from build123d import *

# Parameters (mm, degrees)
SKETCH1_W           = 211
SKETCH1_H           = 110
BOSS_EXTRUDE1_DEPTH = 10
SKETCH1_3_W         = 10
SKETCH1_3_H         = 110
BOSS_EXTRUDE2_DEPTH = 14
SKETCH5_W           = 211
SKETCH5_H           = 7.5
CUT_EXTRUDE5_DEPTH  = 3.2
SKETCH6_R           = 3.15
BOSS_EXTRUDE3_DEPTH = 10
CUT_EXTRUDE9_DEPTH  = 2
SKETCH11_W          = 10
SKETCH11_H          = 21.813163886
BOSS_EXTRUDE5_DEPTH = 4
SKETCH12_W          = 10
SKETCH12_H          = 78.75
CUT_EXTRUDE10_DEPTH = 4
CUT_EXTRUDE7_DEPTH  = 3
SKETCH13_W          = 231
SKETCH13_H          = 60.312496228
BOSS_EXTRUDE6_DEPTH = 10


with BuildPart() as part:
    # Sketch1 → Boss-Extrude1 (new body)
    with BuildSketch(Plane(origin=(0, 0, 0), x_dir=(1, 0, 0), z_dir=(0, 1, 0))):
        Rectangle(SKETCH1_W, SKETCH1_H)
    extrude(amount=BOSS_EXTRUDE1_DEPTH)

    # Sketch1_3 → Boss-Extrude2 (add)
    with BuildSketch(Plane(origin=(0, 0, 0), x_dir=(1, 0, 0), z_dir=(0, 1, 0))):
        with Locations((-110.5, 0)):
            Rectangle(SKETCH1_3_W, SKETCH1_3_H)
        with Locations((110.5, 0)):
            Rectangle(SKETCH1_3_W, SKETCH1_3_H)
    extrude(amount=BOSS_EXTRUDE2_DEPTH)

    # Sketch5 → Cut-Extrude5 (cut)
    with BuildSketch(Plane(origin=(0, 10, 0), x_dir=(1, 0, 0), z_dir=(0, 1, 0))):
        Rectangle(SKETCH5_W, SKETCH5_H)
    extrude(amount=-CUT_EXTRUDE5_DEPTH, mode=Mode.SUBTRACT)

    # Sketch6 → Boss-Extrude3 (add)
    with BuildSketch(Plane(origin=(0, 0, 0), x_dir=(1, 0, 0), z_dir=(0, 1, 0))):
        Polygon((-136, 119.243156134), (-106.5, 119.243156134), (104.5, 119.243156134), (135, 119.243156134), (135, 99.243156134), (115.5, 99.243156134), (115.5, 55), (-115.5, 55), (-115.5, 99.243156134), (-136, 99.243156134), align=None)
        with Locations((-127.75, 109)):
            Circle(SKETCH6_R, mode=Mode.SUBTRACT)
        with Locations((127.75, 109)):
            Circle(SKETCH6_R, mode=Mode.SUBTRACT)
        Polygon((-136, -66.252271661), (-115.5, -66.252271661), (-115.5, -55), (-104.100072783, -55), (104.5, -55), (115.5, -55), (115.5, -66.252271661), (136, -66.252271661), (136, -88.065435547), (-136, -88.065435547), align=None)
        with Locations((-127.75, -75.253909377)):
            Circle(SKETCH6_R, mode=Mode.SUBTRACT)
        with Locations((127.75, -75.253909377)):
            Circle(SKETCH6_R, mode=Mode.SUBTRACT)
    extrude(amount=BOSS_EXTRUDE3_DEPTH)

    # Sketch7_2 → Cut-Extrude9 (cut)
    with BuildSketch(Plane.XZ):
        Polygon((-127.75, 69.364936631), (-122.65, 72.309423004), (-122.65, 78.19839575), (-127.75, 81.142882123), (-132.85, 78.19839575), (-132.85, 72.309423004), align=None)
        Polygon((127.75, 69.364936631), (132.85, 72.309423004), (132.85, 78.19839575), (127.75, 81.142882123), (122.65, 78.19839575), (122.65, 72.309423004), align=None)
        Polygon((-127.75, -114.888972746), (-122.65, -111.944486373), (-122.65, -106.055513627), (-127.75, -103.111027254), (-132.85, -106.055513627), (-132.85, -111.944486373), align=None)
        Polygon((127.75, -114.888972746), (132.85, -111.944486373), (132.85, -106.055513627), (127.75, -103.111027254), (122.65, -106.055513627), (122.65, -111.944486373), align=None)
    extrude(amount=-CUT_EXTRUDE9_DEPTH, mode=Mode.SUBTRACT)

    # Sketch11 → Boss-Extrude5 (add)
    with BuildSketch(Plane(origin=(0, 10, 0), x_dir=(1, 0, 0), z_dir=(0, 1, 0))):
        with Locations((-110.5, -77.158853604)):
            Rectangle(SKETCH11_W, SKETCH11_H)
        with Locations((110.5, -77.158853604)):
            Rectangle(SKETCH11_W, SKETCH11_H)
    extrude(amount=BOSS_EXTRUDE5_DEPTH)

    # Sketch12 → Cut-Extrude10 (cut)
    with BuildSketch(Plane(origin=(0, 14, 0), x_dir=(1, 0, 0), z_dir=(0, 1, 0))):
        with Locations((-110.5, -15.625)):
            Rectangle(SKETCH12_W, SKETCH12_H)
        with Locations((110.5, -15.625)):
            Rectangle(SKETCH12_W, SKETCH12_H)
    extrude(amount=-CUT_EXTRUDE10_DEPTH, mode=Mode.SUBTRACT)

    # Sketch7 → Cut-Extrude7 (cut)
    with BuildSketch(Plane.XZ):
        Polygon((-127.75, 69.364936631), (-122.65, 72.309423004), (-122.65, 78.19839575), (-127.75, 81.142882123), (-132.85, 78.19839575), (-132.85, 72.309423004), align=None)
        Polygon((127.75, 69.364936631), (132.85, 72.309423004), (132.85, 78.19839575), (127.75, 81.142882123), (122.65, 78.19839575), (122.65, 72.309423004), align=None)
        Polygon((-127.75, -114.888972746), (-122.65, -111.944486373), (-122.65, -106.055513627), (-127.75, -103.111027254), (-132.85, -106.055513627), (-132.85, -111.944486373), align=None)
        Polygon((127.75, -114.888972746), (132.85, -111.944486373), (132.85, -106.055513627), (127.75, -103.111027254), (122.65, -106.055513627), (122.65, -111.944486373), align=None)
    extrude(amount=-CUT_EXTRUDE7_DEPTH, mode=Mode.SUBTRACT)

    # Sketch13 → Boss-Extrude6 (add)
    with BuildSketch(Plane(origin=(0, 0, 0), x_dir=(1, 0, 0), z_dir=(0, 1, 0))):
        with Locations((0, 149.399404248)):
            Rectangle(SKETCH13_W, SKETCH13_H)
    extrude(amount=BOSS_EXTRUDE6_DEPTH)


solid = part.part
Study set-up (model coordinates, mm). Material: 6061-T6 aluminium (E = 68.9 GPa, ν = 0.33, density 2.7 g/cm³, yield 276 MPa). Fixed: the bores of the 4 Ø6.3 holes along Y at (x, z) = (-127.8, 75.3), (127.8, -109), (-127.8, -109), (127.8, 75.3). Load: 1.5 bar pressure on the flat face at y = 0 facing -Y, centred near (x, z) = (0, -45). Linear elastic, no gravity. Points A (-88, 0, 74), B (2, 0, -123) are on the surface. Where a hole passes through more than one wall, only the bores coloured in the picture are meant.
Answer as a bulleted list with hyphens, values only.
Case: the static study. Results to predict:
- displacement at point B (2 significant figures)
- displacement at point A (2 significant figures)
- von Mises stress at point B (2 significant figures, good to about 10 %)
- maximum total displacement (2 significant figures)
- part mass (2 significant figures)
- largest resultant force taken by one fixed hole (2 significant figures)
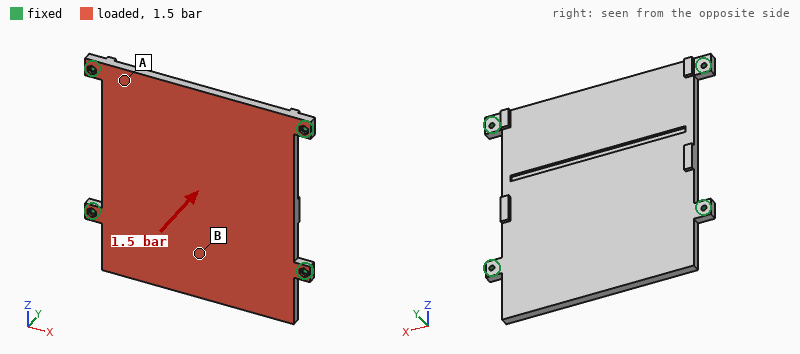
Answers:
- 0.83 mm
- 0.26 mm
- 48 MPa
- 0.98 mm
- 1.7 kg
- 3.8 kN
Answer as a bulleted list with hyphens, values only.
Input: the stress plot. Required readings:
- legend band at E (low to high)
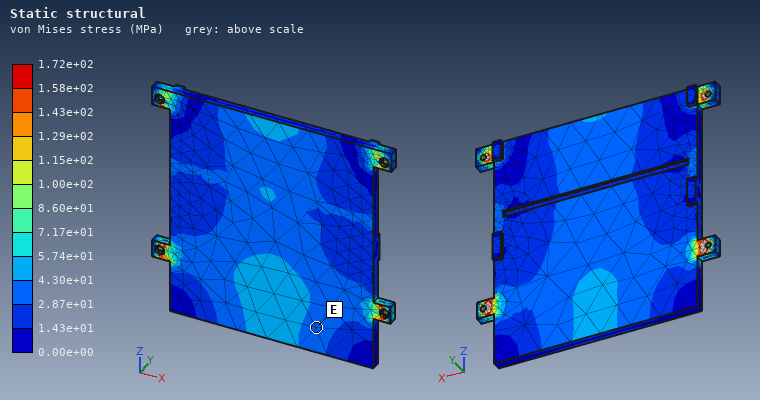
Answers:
- 2.87e+01 to 4.30e+01 MPa
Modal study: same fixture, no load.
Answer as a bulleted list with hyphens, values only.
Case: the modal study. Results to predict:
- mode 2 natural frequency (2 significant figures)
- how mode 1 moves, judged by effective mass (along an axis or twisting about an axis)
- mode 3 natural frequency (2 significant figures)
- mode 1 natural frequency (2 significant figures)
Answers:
- 550 Hz
- along Y
- 1000 Hz
- 470 Hz
